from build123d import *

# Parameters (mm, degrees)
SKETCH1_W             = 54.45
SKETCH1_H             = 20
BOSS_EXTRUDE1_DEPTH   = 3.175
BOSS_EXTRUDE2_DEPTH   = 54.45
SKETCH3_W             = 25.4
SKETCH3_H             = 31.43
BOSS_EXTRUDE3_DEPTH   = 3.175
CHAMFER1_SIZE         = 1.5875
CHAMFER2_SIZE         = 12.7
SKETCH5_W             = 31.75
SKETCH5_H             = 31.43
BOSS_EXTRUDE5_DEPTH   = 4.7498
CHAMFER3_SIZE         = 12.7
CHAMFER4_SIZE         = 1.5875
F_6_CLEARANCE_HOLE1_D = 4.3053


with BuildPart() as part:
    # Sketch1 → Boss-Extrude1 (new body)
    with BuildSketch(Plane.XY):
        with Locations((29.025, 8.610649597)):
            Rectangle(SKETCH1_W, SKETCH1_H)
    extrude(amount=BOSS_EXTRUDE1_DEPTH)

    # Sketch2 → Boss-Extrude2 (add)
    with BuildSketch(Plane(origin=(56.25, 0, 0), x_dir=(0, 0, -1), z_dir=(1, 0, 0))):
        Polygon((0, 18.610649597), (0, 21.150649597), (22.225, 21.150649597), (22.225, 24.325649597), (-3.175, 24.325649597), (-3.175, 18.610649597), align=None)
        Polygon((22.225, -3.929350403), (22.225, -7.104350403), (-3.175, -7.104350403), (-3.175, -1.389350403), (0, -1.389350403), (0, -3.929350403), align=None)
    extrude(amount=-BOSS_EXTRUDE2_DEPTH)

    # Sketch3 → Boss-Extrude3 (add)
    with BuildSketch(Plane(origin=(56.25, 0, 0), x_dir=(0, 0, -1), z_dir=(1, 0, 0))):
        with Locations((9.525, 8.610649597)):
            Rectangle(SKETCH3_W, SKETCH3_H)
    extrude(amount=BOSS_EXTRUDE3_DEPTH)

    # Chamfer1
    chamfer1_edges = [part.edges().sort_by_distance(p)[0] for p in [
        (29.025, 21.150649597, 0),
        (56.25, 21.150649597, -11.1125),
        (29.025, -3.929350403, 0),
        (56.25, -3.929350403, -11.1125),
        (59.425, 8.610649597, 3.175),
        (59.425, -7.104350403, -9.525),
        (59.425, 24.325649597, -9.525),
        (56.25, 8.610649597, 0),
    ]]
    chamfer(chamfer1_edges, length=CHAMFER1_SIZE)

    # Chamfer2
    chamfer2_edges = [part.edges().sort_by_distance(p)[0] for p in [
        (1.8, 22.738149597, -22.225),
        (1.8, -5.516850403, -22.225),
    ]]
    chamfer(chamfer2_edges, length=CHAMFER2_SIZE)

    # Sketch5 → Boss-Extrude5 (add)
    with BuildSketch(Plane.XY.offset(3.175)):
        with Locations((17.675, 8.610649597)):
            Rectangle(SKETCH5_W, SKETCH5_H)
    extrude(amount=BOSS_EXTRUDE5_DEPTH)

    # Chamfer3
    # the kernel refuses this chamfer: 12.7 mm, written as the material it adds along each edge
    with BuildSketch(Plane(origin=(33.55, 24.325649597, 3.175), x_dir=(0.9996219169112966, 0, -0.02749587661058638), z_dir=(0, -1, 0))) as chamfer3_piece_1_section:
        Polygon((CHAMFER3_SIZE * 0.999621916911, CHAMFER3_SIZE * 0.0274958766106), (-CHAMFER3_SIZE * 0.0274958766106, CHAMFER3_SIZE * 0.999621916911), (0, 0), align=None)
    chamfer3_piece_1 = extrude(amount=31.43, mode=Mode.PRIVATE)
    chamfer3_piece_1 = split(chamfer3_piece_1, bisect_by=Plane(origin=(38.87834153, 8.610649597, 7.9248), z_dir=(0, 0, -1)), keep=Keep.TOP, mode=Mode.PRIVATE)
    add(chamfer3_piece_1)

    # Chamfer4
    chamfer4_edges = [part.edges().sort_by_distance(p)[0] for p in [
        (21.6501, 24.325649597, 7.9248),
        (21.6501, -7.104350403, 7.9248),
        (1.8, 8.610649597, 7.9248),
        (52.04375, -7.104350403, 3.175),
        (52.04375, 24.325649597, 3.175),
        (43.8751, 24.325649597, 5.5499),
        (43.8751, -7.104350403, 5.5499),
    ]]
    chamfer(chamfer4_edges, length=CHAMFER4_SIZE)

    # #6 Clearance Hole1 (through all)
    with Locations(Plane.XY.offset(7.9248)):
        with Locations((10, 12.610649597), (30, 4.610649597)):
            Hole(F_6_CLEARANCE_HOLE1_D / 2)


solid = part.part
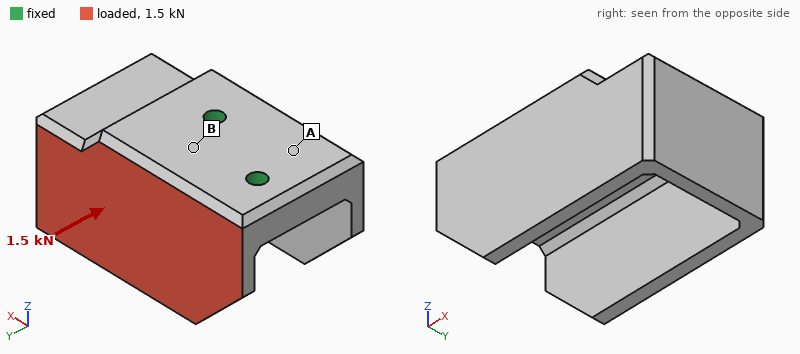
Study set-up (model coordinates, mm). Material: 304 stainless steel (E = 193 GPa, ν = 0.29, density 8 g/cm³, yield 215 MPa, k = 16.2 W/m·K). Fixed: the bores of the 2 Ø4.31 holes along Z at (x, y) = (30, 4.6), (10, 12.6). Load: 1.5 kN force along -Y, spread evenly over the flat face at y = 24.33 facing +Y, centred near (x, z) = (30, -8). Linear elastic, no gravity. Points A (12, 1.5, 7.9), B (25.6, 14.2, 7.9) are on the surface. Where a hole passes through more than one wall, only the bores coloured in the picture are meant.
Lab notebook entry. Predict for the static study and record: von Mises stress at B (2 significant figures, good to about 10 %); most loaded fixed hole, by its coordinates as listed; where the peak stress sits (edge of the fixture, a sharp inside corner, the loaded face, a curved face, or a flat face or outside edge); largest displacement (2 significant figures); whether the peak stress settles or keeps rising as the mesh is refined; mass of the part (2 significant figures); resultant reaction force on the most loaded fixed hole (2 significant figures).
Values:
26 MPa
(30, 4.6)
edge of the fixture
62 µm
keeps rising
170 g
1.3 kN
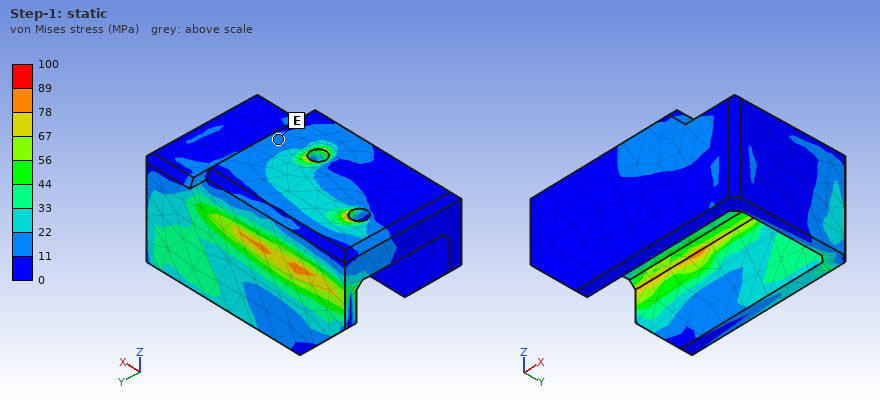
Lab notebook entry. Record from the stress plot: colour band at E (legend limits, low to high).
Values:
11 to 22 MPa
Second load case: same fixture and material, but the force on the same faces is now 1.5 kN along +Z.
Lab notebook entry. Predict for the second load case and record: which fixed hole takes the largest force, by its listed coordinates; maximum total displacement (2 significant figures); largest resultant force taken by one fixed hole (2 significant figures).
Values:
(30, 4.6)
36 µm
910 N
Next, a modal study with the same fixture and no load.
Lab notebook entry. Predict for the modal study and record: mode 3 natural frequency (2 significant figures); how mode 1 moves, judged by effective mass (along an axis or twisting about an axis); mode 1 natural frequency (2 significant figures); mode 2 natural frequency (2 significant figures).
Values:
6000 Hz
along Y
3900 Hz
5900 Hz
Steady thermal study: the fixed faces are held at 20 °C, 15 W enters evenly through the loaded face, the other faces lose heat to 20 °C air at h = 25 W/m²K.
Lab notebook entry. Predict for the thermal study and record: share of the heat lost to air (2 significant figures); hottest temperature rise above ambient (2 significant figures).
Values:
30 %
67 K
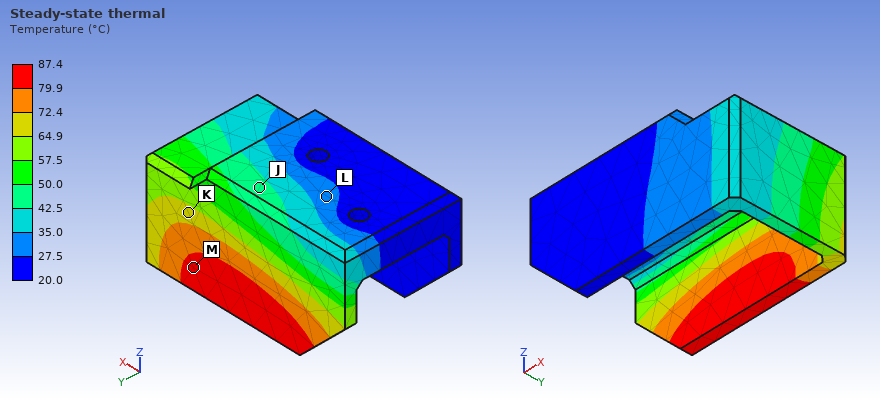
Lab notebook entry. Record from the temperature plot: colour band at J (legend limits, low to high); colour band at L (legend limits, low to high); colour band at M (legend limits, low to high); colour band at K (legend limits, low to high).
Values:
42.5 to 50.0 °C
27.5 to 35.0 °C
79.9 to 87.4 °C
64.9 to 72.4 °C
